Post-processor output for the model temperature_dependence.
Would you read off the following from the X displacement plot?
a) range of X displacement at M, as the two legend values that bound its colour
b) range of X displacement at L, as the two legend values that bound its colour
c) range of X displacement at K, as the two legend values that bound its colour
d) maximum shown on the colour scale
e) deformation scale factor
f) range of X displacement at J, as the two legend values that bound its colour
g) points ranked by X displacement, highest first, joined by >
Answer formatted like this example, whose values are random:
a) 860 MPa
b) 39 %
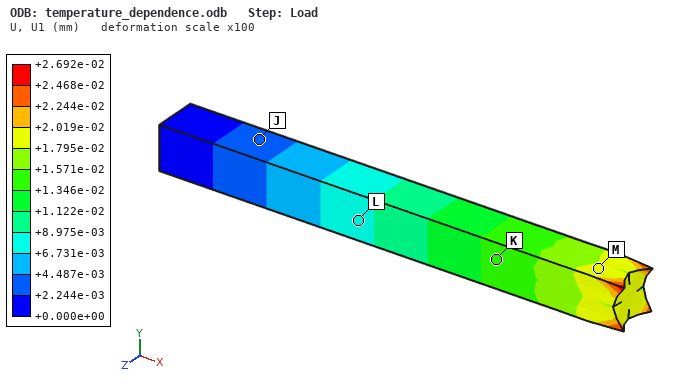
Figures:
a) +1.795e-02 to +2.019e-02 mm
b) +6.731e-03 to +8.975e-03 mm
c) +1.346e-02 to +1.571e-02 mm
d) +2.692e-02 mm
e) 100
f) +2.244e-03 to +4.487e-03 mm
g) M > K > L > J
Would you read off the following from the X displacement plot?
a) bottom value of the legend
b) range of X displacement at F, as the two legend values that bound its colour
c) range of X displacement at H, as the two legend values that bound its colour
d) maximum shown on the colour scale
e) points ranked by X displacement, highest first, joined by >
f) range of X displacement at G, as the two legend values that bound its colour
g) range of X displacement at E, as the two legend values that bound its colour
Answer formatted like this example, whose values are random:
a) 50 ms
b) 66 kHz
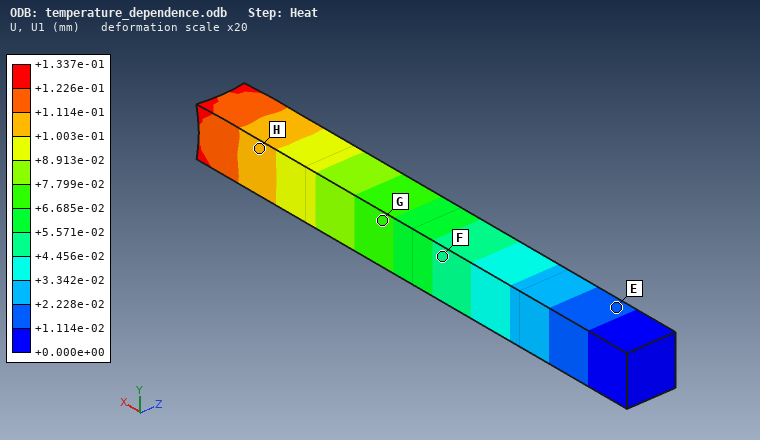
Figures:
a) +0.000e+00 mm
b) +4.456e-02 to +5.571e-02 mm
c) +1.003e-01 to +1.114e-01 mm
d) +1.337e-01 mm
e) H > G > F > E
f) +6.685e-02 to +7.799e-02 mm
g) +1.114e-02 to +2.228e-02 mm
